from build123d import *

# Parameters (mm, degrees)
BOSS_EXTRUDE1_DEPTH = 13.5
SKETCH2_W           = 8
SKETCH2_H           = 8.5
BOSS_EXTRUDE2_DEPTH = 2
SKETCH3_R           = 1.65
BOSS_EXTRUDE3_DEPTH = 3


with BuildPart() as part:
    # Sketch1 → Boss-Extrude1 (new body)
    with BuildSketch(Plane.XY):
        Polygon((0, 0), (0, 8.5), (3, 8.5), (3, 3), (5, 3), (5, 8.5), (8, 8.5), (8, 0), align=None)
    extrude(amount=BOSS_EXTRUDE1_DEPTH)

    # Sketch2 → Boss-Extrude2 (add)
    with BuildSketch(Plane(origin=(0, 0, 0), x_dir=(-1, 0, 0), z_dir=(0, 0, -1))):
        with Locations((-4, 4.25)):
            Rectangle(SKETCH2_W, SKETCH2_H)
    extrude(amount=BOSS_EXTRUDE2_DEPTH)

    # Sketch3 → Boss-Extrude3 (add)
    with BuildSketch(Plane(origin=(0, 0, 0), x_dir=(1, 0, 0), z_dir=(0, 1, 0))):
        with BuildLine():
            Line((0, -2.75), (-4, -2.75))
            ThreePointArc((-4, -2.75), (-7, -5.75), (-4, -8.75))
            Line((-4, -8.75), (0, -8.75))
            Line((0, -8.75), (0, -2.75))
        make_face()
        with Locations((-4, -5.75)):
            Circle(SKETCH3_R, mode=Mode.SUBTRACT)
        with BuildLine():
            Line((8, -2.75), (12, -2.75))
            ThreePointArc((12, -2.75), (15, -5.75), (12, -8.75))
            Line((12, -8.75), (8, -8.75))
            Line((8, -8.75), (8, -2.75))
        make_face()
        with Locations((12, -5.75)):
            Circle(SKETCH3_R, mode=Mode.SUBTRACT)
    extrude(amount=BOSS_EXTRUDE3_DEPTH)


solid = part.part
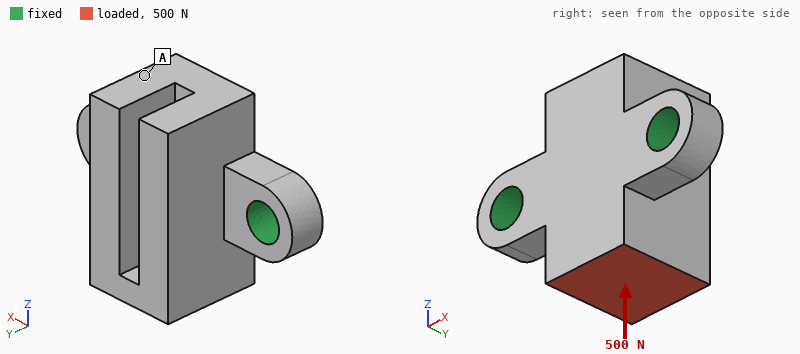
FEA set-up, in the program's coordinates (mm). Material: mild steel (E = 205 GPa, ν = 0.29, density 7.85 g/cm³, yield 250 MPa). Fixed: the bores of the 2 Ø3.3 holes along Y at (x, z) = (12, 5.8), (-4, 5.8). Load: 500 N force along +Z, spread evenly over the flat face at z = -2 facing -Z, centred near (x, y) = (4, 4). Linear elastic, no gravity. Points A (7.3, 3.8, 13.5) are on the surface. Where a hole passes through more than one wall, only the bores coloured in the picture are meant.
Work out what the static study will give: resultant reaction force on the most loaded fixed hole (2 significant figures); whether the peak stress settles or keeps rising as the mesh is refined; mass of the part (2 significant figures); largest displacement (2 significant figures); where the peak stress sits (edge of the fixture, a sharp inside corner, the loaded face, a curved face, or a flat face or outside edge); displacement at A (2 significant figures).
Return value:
250 N
keeps rising
8.5 g
8.8 µm
edge of the fixture
6.2 µm
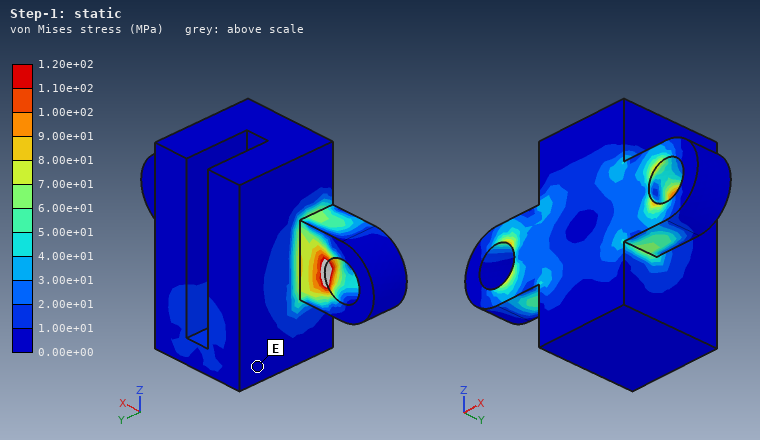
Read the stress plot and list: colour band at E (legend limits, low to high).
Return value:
0.00e+00 to 1.00e+01 MPa
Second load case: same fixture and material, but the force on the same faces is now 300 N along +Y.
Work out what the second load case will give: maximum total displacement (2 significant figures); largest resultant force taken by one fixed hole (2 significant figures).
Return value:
14 µm
160 N
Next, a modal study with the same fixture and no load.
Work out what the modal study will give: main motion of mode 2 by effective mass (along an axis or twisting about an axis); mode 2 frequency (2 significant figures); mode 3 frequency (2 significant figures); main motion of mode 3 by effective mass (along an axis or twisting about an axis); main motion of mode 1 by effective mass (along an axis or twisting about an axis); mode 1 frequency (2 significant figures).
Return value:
along Y
31 kHz
37 kHz
along X
along Z
14 kHz
